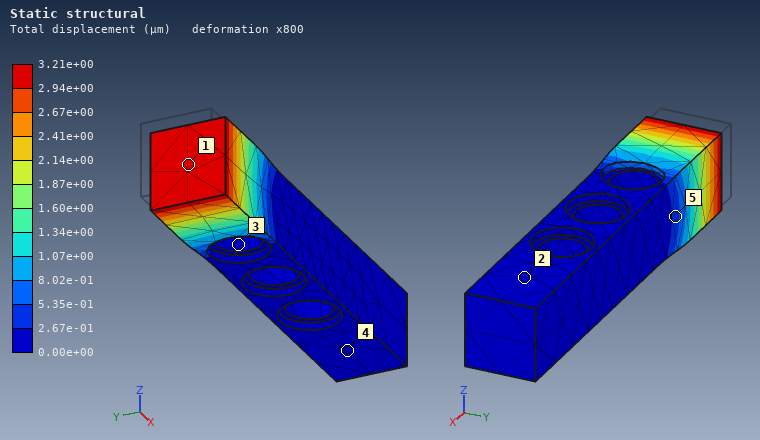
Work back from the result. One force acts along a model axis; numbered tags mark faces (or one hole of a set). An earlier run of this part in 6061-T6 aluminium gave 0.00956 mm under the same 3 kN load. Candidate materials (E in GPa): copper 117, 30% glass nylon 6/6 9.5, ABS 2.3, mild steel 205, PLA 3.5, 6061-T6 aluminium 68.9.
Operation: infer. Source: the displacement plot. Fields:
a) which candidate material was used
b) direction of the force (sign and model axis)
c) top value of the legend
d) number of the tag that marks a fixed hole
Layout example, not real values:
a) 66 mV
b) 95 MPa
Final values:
a) mild steel
b) +X
c) 3.21e+00 µm
d) 3
